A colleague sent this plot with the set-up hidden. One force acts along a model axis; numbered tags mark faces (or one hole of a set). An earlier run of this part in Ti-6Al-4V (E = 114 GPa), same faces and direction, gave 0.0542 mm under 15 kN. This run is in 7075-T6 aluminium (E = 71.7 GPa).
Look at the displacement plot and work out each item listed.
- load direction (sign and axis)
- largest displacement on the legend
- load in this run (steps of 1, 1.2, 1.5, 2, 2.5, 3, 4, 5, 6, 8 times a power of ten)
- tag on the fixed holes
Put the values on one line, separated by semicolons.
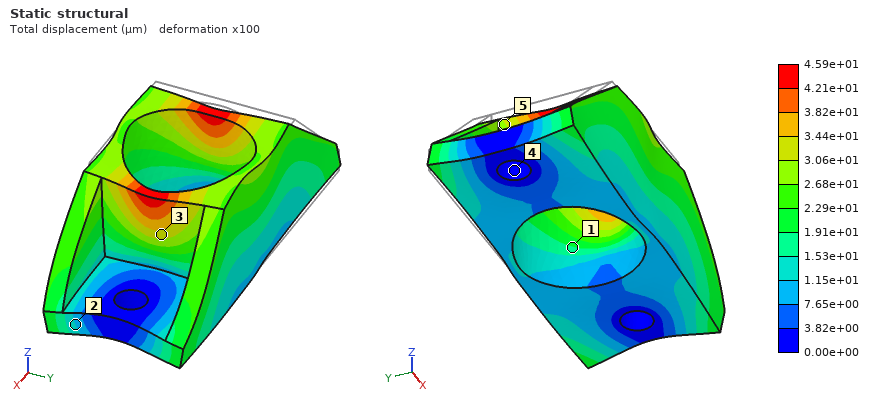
+X; 4.59e+01 µm; 8 kN; 4
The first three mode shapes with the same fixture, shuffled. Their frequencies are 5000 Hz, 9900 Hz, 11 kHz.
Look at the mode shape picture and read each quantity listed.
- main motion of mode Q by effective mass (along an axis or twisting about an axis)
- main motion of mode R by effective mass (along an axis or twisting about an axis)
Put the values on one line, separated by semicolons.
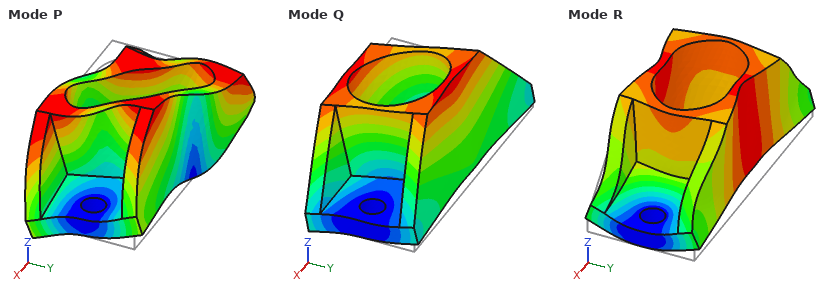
along Y; along Z
